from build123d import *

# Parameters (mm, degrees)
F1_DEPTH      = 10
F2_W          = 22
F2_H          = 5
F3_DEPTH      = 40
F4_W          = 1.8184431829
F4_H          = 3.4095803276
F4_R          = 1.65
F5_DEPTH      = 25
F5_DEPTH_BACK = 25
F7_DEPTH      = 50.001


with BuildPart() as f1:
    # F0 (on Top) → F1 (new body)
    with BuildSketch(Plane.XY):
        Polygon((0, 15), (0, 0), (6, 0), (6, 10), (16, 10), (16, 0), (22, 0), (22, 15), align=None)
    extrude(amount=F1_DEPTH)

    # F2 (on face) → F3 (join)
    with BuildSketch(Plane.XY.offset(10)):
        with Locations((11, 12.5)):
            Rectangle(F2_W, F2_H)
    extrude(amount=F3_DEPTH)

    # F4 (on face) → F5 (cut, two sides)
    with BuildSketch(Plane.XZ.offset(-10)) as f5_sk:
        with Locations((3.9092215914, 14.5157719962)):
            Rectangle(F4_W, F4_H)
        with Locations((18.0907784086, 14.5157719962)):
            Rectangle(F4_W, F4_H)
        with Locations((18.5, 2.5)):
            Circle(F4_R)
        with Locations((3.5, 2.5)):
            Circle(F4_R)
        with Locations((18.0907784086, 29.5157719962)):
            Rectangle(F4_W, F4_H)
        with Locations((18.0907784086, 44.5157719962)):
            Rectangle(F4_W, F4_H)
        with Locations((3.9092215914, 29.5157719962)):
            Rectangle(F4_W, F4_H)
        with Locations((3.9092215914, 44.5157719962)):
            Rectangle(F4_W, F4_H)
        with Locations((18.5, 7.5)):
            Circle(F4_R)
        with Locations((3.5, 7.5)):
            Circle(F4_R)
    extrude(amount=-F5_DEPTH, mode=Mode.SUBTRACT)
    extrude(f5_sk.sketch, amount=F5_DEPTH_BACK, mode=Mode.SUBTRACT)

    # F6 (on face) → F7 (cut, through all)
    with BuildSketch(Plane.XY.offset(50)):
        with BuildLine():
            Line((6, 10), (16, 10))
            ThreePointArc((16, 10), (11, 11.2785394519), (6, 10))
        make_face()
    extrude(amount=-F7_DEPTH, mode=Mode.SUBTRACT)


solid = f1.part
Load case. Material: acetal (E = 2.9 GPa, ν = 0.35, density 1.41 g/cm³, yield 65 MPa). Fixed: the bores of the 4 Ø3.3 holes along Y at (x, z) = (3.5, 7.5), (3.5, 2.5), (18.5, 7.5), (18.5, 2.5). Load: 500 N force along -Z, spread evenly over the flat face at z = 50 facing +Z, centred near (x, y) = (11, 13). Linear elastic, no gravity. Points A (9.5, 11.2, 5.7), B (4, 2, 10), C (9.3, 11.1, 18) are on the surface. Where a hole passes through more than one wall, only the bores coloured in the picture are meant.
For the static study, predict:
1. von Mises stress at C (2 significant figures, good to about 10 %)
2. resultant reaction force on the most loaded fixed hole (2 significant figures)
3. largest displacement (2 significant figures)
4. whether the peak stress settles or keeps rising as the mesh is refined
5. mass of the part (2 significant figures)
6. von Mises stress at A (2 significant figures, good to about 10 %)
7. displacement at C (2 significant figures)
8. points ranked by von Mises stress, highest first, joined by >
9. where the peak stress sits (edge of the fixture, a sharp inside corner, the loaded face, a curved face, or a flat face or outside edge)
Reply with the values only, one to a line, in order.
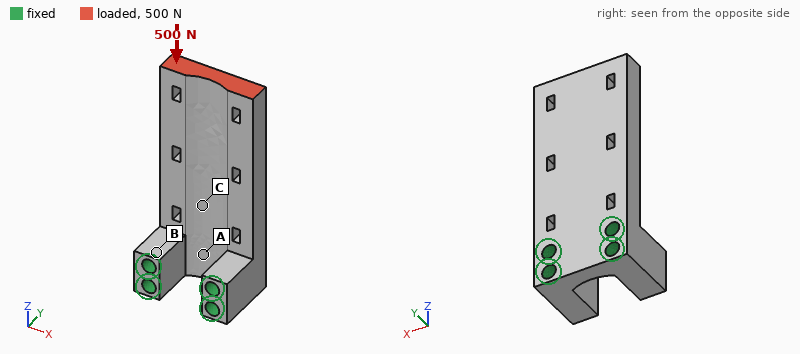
5.2 MPa
210 N
84 µm
keeps rising
7.9 g
1.8 MPa
20 µm
C > A > B
edge of the fixture
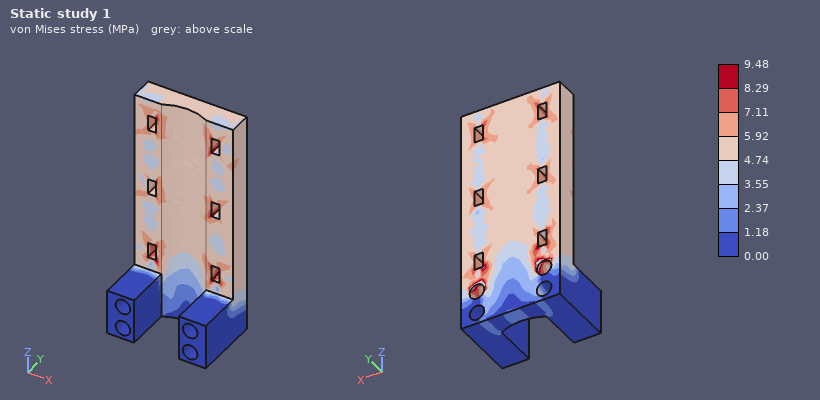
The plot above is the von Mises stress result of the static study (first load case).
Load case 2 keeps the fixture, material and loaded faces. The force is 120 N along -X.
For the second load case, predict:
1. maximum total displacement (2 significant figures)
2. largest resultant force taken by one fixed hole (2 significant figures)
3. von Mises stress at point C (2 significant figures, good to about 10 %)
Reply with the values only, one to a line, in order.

0.35 mm
280 N
5.1 MPa
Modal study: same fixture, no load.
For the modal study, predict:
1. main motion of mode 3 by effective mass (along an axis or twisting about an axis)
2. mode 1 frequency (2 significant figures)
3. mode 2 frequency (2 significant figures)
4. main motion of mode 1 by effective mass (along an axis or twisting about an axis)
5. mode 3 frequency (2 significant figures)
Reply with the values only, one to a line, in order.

along X
620 Hz
2100 Hz
along Y
2400 Hz
